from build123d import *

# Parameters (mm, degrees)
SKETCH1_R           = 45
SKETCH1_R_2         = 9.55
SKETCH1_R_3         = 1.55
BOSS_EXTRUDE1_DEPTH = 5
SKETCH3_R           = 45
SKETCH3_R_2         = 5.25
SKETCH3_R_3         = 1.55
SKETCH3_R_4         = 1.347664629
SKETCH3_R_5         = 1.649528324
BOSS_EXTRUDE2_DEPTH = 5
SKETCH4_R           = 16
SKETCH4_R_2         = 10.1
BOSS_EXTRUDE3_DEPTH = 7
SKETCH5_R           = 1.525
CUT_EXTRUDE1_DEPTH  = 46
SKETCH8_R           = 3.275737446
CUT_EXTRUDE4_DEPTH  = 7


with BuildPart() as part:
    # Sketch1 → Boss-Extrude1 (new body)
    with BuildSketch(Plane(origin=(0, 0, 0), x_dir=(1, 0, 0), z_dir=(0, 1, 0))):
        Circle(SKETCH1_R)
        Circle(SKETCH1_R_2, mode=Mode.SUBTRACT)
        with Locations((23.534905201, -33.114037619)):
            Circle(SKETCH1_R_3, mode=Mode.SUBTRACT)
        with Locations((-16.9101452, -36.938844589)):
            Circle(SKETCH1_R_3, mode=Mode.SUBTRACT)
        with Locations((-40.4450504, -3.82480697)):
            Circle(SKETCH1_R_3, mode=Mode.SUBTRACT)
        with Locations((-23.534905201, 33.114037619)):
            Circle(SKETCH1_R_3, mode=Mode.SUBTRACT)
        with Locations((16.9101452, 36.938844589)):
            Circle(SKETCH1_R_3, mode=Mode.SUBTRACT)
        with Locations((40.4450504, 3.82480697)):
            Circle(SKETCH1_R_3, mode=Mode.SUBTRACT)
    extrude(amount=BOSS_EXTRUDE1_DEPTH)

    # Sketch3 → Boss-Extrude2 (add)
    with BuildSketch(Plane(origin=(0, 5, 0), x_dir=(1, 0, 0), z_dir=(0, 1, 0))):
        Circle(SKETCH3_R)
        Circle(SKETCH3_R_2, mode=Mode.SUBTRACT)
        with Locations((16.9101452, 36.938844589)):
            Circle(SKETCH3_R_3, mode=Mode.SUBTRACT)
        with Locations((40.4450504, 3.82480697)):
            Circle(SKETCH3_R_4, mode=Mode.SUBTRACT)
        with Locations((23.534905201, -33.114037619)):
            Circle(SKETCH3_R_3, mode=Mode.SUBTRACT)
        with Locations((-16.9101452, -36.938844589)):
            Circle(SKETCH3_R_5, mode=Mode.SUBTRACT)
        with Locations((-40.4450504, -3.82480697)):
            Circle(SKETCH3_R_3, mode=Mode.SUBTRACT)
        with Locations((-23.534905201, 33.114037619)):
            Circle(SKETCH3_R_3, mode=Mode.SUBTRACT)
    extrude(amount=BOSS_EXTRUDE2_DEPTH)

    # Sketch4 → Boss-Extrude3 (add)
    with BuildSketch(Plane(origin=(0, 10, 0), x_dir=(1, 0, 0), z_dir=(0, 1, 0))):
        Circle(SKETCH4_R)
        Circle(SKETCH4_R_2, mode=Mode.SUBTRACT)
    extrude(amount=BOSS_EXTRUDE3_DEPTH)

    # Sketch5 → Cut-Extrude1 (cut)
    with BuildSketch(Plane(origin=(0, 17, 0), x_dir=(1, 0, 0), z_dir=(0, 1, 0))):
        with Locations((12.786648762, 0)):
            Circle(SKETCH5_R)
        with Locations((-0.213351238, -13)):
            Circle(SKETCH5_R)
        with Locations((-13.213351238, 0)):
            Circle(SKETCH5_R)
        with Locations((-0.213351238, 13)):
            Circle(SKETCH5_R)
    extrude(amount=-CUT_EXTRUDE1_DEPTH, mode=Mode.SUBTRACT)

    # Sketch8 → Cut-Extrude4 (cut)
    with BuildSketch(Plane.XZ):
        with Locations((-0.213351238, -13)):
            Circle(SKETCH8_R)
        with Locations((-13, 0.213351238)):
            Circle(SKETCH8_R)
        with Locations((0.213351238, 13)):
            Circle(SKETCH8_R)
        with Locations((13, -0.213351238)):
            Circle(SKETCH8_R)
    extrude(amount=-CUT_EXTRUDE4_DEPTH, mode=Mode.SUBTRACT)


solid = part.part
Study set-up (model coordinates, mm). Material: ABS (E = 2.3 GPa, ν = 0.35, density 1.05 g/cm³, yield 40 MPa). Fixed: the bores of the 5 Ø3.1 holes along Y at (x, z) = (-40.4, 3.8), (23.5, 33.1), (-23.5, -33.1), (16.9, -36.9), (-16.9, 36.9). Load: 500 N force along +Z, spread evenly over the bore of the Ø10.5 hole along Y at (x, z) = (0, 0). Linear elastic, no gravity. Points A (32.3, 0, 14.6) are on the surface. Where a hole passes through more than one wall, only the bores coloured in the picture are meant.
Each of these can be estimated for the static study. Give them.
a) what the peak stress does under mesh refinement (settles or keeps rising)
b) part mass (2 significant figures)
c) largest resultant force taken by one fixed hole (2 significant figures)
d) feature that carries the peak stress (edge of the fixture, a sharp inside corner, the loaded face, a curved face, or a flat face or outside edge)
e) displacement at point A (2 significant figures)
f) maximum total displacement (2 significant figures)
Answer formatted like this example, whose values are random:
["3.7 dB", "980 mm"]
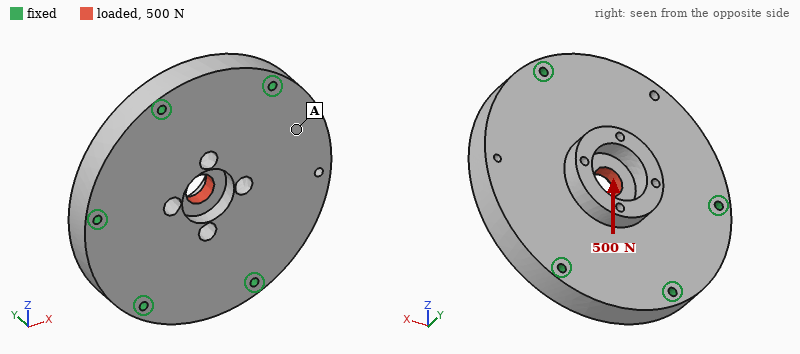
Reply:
["keeps rising", "67 g", "130 N", "edge of the fixture", "3.9 µm", "23 µm"]
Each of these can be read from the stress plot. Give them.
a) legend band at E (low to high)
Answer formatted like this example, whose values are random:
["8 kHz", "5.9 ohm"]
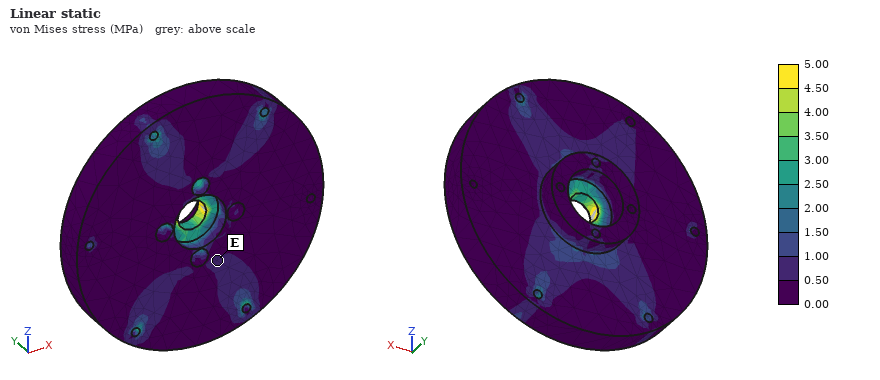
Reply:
["0.50 to 1.00 MPa"]
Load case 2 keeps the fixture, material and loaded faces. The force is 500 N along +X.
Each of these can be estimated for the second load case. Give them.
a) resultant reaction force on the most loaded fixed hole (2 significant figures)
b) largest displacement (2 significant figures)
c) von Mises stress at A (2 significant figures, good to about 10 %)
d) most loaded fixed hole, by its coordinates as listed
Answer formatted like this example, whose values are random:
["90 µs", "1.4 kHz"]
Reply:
["150 N", "28 µm", "0.44 MPa", "(-40.4, 3.8)"]
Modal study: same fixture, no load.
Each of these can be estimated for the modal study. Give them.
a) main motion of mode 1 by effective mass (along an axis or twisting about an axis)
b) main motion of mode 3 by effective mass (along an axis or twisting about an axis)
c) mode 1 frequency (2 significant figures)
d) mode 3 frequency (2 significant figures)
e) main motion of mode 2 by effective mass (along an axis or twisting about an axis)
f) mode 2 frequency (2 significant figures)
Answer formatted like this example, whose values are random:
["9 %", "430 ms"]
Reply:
["along Y", "twisting about X", "1900 Hz", "4800 Hz", "along Y", "2900 Hz"]
